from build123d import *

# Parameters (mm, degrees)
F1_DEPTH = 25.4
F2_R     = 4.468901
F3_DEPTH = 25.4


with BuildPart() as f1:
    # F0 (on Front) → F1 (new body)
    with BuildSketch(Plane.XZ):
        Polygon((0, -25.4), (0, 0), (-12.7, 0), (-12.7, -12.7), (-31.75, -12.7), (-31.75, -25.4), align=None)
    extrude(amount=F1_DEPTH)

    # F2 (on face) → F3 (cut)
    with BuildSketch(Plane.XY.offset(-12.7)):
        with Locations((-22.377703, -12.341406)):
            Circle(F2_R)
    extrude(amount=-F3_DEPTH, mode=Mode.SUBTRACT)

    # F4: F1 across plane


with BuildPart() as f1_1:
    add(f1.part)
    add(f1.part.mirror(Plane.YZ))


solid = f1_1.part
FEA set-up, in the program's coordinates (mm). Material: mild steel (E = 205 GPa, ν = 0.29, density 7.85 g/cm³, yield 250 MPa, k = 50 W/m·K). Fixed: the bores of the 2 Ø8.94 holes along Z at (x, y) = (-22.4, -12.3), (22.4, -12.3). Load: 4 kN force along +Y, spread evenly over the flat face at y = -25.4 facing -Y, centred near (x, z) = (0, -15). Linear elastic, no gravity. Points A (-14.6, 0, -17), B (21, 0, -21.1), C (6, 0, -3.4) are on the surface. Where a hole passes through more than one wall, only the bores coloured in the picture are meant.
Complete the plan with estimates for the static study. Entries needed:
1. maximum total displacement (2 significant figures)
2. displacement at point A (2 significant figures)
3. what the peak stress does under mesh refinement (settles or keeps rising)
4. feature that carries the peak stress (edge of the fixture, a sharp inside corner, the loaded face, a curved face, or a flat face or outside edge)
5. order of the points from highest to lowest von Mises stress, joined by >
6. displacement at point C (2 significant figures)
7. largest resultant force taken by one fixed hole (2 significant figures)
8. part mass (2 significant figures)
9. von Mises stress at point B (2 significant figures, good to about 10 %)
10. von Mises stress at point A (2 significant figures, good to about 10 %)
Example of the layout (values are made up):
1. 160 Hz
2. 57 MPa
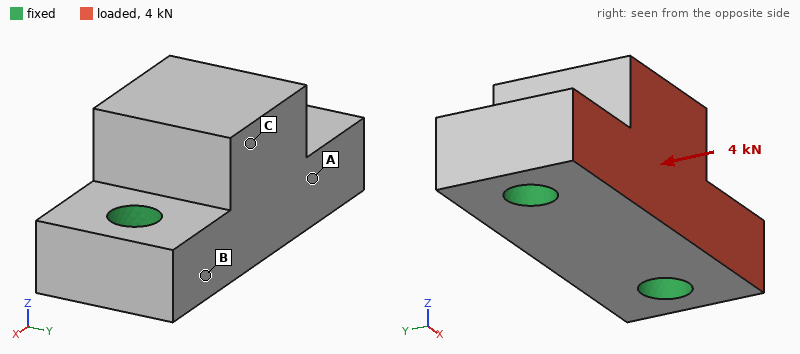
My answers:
1. 3.1 µm
2. 0.88 µm
3. keeps rising
4. edge of the fixture
5. A > B > C
6. 2.5 µm
7. 2.0 kN
8. 210 g
9. 5.5 MPa
10. 9.9 MPa
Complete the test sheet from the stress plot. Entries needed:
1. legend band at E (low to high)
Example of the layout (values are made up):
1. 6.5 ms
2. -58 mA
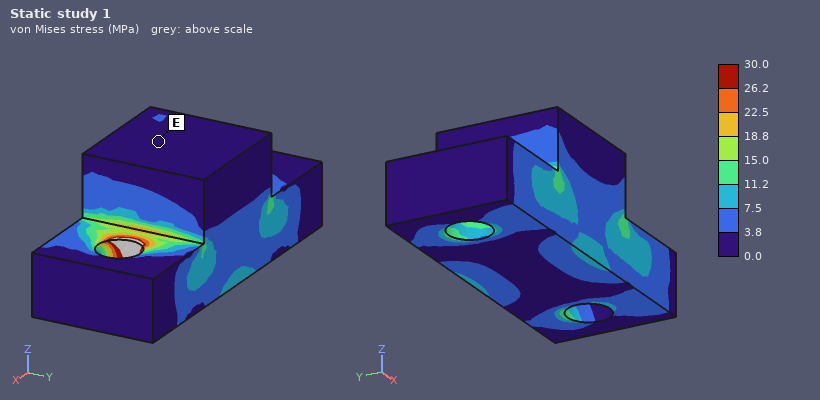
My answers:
1. 0.0 to 3.8 MPa
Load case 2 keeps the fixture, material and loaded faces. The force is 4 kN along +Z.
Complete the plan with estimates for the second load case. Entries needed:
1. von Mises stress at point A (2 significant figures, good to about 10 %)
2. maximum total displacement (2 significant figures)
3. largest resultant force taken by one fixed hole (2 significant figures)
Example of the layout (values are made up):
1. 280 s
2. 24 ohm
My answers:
1. 15 MPa
2. 5.9 µm
3. 2.0 kN
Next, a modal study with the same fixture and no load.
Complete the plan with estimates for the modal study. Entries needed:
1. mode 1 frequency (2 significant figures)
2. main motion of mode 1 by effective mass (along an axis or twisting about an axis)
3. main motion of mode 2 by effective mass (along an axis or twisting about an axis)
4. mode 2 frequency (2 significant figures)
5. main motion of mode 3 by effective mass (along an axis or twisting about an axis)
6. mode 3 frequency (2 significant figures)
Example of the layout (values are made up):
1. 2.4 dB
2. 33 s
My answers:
1. 14 kHz
2. along Y
3. along Z
4. 22 kHz
5. along X
6. 27 kHz
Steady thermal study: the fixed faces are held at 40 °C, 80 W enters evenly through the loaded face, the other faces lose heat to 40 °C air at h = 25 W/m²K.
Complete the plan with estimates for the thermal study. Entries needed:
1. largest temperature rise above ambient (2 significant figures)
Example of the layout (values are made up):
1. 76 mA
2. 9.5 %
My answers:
1. 39 K
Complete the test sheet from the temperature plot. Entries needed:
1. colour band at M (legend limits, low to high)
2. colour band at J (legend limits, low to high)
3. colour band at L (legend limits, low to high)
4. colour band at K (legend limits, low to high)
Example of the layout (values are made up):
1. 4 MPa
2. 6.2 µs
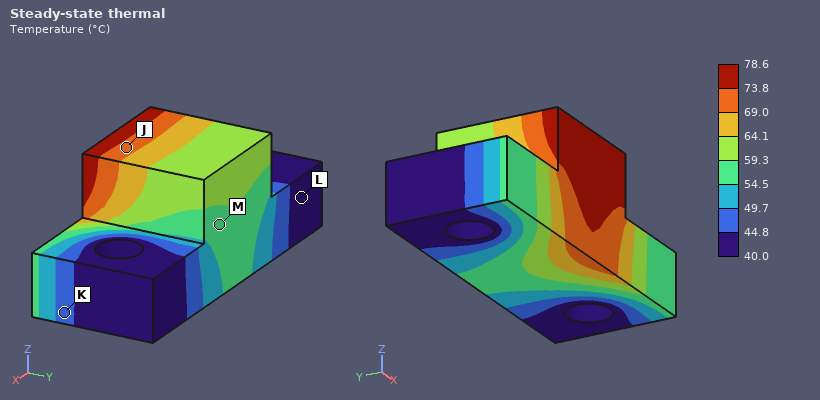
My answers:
1. 54.5 to 59.3 °C
2. 69.0 to 73.8 °C
3. 40.0 to 44.8 °C
4. 44.8 to 49.7 °C
